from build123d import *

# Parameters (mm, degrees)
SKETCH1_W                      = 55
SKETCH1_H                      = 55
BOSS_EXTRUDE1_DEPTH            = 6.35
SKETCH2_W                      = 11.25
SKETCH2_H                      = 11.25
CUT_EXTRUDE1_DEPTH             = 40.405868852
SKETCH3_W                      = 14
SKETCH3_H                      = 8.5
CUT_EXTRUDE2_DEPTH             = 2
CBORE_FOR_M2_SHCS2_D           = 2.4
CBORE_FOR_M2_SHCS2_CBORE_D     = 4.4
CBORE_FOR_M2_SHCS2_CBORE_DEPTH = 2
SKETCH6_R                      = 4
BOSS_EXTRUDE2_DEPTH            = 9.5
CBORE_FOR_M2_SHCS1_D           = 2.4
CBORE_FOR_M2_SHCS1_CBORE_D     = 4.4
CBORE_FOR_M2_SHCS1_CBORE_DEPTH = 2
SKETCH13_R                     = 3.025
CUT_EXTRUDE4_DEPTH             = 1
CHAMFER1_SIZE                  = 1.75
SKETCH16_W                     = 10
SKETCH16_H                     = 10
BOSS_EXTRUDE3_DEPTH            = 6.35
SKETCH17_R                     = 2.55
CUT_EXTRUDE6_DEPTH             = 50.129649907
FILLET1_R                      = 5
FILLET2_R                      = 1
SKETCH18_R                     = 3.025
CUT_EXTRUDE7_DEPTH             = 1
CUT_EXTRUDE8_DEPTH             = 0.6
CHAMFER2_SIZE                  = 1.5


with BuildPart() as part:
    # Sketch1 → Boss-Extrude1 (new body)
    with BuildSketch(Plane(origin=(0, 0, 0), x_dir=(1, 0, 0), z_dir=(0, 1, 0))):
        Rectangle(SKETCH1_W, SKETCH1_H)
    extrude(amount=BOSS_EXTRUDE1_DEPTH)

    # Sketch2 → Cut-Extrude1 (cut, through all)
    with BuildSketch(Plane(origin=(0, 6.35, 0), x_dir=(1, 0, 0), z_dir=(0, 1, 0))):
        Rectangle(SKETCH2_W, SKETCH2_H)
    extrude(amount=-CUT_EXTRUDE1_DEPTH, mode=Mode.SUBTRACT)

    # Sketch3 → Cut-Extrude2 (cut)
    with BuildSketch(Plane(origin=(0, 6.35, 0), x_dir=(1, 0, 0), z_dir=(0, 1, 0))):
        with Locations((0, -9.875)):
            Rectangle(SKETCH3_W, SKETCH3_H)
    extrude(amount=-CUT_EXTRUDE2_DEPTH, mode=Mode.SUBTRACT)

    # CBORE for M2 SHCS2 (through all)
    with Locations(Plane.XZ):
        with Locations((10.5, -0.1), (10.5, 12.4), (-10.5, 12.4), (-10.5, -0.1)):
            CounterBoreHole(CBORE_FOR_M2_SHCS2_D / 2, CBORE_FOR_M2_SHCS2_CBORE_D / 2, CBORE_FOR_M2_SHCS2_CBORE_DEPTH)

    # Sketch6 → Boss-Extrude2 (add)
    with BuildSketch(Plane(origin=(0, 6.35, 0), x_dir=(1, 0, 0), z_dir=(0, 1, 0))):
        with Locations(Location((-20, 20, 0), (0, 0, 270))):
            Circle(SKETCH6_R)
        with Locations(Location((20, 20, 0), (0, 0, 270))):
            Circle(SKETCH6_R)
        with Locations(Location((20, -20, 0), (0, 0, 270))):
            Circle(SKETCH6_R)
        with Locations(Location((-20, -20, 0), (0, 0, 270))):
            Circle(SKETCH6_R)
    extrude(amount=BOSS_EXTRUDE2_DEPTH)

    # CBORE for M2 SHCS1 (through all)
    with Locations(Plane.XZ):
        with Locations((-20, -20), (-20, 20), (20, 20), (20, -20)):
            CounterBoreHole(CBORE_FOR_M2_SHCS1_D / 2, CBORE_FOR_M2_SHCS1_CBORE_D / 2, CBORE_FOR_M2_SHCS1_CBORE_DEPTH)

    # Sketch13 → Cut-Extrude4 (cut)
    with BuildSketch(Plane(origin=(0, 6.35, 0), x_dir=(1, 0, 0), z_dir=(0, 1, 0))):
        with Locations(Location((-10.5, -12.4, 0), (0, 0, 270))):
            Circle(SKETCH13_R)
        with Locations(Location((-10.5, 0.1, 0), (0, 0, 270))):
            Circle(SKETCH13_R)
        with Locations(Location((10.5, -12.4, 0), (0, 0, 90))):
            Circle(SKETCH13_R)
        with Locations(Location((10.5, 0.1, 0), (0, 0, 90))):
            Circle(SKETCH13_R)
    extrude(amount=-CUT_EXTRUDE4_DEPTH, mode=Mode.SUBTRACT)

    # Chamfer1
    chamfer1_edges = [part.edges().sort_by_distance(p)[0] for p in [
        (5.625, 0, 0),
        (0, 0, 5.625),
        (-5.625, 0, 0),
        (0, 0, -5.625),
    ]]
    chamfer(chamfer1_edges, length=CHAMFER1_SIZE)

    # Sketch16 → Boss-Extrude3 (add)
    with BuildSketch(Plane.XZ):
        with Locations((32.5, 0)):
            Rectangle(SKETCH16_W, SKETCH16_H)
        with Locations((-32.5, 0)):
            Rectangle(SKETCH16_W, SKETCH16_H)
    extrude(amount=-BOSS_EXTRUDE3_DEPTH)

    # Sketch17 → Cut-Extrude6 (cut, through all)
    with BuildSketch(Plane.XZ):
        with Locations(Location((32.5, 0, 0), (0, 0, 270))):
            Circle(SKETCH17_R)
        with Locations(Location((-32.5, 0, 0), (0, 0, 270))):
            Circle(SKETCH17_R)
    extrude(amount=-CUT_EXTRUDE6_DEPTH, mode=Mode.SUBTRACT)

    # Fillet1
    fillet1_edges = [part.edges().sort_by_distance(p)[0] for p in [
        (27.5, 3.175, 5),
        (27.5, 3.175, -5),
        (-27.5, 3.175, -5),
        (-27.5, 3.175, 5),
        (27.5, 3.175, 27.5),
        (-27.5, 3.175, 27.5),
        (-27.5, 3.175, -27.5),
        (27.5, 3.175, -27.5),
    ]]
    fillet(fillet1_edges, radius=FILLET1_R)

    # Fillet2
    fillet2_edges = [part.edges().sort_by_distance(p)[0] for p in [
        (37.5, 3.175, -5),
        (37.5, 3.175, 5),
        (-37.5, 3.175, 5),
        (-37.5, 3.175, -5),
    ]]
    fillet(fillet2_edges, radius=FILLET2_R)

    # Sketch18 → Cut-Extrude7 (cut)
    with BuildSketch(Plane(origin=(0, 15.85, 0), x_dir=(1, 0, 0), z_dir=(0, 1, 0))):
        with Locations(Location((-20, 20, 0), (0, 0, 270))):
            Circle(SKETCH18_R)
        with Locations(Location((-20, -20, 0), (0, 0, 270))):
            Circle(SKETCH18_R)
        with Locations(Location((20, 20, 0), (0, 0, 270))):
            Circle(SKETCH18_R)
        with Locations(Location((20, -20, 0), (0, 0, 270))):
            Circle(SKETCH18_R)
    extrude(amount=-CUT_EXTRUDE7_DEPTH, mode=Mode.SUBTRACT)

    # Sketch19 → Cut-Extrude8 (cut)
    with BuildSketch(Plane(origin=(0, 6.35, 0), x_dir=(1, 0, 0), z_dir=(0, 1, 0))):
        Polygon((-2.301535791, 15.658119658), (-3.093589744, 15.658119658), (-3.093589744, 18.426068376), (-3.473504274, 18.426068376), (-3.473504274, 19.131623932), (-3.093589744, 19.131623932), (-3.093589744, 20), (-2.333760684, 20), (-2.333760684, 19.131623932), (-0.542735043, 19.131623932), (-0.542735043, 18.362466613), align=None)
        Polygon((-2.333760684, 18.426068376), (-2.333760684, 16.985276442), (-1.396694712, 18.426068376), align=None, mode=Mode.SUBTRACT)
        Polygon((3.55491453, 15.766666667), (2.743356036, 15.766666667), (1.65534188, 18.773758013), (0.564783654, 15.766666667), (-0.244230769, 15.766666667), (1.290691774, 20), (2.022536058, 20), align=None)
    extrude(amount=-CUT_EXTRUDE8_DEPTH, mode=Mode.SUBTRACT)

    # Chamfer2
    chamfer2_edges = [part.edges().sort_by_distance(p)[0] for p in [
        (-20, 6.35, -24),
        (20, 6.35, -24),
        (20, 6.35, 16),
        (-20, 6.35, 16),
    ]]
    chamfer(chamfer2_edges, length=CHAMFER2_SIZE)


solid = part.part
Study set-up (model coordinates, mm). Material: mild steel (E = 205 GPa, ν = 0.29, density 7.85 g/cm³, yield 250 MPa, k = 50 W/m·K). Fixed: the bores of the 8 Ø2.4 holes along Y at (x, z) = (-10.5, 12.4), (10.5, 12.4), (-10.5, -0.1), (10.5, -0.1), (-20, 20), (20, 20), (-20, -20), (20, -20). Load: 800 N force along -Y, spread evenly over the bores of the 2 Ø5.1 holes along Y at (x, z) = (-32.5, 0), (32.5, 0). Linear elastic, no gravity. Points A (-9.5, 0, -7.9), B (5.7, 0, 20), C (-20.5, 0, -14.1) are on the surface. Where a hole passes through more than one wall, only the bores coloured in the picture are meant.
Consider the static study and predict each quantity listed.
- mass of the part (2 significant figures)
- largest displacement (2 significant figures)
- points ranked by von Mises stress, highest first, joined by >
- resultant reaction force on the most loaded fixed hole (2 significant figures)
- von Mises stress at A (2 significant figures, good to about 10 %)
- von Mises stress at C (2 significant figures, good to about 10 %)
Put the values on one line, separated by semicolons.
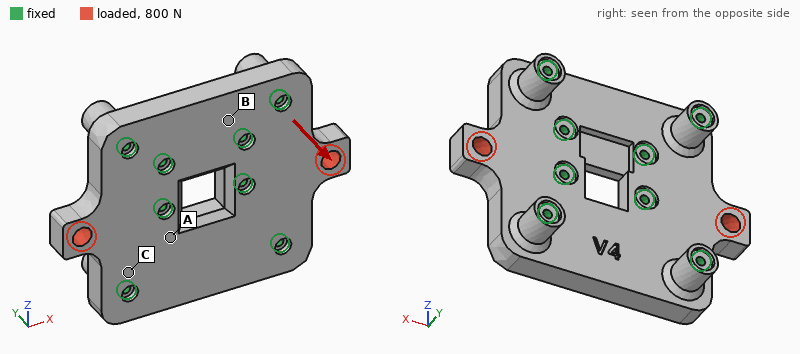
160 g; 13 µm; C > A > B; 290 N; 8.4 MPa; 17 MPa
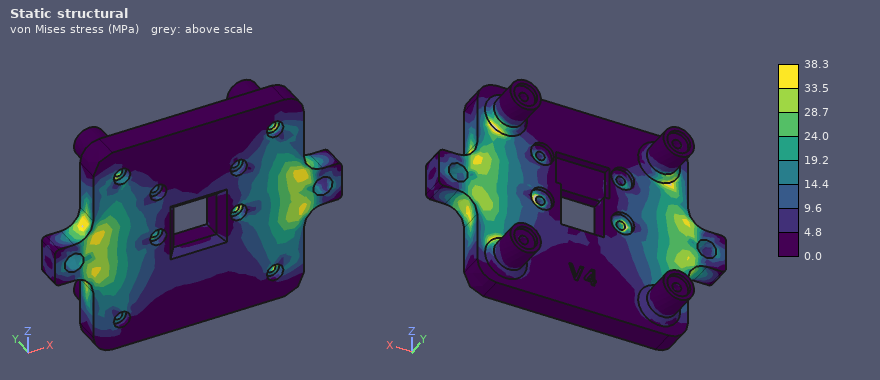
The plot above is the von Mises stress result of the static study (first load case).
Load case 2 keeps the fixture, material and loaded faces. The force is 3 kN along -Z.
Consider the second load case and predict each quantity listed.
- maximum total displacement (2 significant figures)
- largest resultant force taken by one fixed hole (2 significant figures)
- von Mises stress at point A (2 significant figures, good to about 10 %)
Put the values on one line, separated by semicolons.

7.7 µm; 680 N; 6.3 MPa
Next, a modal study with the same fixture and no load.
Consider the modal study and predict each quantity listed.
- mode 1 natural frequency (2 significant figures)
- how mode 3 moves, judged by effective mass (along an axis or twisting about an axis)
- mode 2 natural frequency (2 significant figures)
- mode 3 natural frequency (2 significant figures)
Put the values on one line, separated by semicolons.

14 kHz; along Y; 14 kHz; 20 kHz
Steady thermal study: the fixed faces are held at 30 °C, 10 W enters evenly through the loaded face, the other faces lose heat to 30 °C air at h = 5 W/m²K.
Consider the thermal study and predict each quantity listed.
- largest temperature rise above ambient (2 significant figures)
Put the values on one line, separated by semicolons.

22 K
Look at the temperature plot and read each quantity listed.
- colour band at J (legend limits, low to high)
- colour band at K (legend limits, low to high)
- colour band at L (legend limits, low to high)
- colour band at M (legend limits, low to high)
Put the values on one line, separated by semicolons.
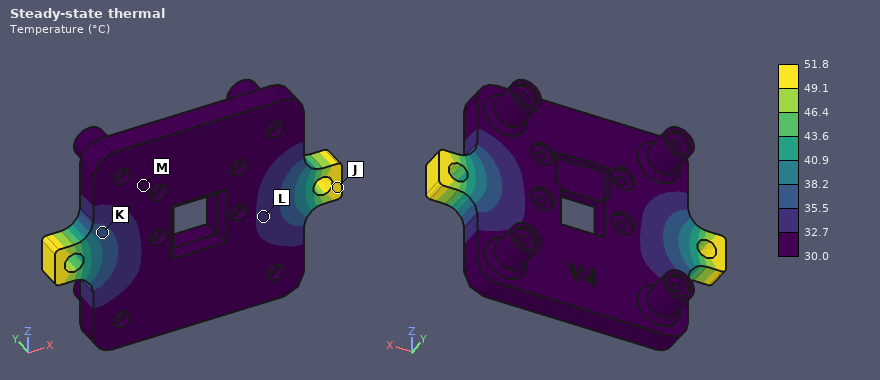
49.1 to 51.8 °C; 35.5 to 38.2 °C; 32.7 to 35.5 °C; 30.0 to 32.7 °C
